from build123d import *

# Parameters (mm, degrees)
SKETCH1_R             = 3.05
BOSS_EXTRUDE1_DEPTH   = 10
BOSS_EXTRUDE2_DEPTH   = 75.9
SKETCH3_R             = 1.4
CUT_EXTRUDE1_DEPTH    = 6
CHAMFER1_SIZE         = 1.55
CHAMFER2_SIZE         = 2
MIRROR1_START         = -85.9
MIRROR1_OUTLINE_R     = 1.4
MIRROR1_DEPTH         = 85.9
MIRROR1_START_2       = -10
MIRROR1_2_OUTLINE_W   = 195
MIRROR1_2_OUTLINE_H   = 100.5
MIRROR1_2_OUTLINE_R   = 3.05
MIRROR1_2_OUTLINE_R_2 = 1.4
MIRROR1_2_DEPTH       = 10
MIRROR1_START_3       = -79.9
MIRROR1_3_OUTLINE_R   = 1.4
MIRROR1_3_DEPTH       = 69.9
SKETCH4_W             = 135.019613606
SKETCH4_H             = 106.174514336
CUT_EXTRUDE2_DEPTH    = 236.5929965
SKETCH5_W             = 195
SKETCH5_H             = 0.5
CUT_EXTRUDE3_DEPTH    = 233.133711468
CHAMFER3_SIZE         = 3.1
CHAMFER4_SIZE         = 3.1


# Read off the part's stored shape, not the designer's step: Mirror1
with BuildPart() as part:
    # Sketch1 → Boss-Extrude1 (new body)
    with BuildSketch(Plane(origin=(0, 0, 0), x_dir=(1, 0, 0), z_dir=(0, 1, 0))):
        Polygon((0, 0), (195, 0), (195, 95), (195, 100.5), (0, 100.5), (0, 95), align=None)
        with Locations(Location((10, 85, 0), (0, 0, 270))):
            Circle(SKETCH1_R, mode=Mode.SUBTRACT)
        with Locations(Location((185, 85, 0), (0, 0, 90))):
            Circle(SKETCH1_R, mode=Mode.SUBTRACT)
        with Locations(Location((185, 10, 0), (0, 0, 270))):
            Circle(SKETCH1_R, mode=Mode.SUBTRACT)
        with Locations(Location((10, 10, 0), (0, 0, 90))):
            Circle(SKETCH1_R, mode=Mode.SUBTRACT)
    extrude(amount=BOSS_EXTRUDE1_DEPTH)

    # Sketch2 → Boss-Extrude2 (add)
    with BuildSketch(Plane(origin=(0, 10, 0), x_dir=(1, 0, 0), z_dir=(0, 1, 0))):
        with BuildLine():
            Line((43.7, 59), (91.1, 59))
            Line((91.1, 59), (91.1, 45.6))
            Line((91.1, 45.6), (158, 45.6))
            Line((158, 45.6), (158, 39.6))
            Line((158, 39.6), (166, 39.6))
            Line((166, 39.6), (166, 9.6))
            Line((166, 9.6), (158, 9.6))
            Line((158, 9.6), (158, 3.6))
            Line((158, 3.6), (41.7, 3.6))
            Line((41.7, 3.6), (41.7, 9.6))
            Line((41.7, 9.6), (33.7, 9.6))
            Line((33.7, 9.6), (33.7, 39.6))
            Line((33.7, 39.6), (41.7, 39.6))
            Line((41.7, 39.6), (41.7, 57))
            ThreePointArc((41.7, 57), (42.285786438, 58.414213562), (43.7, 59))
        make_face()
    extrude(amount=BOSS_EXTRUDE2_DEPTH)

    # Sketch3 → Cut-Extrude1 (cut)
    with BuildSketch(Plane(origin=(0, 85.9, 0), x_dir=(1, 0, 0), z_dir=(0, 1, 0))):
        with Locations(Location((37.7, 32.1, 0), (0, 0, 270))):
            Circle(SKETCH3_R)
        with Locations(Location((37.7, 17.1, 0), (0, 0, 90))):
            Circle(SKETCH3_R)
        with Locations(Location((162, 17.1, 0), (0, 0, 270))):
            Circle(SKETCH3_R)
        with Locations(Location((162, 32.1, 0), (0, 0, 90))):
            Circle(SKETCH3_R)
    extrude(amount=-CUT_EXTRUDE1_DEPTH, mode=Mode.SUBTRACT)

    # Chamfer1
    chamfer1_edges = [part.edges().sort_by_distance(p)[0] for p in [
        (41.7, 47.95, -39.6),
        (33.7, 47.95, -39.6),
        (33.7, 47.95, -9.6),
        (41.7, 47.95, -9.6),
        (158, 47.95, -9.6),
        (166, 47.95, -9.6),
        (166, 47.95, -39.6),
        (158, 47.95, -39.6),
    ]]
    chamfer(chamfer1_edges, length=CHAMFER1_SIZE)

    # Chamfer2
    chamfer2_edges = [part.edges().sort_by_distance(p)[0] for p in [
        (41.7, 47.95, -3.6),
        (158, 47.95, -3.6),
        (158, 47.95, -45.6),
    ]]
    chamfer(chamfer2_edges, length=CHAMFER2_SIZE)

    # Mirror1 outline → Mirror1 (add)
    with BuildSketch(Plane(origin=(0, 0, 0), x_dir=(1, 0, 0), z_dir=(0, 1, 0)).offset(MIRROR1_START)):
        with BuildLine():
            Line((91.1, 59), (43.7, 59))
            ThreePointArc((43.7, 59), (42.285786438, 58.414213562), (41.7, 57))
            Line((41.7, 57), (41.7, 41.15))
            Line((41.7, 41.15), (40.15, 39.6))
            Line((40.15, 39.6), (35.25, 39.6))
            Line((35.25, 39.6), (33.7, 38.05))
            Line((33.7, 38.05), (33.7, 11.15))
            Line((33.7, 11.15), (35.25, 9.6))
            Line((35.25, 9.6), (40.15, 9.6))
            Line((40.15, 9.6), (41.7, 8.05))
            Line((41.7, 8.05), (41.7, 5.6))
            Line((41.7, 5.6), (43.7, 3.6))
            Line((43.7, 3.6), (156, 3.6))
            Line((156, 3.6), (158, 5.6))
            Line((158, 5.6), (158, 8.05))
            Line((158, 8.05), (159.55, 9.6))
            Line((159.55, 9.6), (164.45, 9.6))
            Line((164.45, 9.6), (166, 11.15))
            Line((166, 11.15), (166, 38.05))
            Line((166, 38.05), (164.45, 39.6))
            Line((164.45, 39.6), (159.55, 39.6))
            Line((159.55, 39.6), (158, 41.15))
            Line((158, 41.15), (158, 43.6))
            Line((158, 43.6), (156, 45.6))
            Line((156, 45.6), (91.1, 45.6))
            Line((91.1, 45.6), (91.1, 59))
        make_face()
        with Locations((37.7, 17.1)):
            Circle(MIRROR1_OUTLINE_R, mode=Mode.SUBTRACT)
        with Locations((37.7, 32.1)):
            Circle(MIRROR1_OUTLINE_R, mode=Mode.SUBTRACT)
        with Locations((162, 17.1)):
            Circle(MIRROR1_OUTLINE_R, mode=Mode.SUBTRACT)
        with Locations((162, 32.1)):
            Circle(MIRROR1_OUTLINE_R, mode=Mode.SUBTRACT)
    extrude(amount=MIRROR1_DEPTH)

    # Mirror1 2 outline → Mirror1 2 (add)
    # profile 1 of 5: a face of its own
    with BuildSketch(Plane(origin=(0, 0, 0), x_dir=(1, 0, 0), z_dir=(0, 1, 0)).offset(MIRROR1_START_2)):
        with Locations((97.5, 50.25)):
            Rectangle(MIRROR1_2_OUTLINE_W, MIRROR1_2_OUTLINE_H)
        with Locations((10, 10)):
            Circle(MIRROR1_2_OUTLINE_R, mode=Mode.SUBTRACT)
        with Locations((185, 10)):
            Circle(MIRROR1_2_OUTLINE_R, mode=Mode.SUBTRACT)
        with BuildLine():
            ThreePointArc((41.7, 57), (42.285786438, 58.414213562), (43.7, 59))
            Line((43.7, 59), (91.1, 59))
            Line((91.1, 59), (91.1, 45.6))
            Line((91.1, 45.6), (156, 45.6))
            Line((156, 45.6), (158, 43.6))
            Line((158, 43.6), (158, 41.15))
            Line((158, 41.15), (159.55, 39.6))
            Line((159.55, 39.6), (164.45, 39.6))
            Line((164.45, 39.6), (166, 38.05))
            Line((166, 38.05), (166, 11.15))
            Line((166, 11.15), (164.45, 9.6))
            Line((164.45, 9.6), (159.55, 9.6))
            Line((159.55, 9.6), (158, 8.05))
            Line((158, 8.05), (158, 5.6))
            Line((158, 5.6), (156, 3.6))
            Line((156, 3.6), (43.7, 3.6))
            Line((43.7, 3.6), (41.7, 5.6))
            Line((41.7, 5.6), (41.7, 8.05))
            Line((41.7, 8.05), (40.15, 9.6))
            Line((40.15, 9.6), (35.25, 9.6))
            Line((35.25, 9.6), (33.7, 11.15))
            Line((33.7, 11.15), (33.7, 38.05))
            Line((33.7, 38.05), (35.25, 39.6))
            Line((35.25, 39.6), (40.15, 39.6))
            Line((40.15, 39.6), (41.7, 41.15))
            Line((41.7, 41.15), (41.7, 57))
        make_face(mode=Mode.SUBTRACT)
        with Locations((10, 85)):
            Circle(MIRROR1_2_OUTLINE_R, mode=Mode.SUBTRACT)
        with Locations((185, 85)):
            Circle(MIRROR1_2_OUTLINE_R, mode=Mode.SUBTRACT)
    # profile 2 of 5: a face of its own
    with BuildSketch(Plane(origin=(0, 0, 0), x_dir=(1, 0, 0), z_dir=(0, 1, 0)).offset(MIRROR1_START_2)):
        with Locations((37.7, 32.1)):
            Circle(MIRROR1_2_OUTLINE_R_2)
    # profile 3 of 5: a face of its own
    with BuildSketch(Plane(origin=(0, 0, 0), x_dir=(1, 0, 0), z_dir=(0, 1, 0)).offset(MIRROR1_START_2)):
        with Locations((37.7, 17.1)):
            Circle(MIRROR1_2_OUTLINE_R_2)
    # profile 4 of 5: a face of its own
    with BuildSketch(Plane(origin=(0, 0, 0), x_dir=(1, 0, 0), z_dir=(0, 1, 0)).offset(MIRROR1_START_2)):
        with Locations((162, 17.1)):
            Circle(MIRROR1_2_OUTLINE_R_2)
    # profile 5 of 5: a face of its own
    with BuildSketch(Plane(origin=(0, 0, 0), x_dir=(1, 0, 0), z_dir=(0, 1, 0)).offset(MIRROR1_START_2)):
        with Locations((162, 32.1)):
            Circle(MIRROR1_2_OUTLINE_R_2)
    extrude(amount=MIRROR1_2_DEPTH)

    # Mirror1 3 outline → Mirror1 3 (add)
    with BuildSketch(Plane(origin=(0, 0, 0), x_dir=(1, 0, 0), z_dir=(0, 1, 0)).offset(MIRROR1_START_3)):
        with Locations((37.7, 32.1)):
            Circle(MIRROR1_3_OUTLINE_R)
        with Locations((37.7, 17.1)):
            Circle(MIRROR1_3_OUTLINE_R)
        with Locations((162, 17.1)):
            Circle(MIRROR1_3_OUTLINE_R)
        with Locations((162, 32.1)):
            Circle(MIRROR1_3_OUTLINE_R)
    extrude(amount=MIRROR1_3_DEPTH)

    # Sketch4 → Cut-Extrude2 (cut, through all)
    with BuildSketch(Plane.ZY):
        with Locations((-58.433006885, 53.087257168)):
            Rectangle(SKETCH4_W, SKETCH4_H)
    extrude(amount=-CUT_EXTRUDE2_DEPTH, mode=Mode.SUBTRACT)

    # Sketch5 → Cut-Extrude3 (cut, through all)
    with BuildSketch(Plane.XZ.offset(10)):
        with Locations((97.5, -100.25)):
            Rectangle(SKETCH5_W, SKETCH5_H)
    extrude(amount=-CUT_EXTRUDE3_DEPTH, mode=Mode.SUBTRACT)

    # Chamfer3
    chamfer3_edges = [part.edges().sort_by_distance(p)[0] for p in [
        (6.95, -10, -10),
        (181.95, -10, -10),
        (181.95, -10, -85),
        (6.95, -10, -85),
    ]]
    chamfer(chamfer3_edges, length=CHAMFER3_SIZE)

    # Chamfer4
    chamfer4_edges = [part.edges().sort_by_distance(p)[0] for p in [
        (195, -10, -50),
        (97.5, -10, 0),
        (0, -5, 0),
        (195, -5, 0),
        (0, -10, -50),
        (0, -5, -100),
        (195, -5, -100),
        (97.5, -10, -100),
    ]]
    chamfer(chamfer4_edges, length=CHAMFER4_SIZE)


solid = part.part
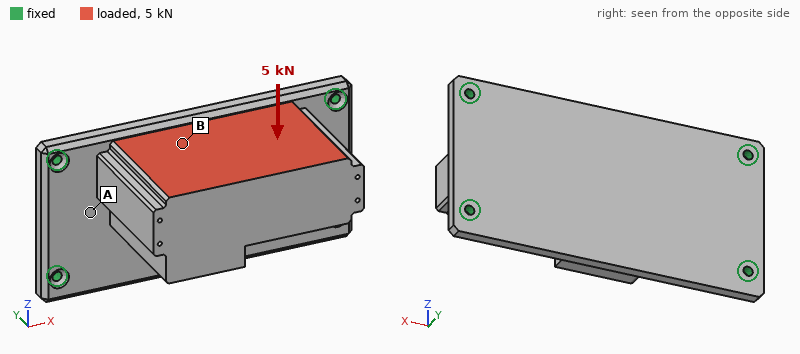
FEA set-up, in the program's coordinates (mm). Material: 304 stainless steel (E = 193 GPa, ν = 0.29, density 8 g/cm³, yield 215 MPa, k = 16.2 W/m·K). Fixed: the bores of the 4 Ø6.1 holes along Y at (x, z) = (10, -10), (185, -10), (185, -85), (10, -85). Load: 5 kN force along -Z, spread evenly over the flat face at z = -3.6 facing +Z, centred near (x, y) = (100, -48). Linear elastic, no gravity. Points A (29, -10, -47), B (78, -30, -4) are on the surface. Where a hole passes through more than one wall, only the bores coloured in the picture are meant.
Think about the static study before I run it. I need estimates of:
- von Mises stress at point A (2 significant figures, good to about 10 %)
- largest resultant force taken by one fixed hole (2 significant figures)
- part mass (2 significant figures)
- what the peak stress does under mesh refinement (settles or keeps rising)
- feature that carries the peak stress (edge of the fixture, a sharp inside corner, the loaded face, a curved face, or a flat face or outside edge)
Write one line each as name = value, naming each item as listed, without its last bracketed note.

von Mises stress at point A = 32 MPa
largest resultant force taken by one fixed hole = 2.6 kN
part mass = 5.2 kg
what the peak stress does under mesh refinement = keeps rising
feature that carries the peak stress = edge of the fixture
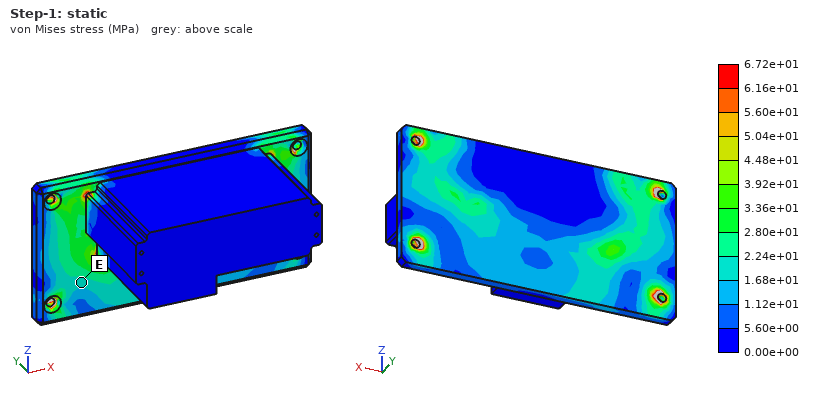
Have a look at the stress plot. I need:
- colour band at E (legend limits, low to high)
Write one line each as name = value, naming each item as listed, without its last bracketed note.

colour band at E = 1.68e+01 to 2.24e+01 MPa
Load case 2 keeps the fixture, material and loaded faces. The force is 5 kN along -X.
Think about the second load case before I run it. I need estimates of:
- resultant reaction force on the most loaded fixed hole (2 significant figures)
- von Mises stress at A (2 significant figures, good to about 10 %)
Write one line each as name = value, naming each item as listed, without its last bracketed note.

resultant reaction force on the most loaded fixed hole = 2.0 kN
von Mises stress at A = 8.3 MPa
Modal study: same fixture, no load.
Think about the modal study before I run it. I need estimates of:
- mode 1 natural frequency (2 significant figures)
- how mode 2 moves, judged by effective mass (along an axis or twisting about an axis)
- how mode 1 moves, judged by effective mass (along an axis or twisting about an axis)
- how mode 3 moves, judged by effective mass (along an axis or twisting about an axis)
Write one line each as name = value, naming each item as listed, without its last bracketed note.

mode 1 natural frequency = 840 Hz
how mode 2 moves, judged by effective mass = along Y
how mode 1 moves, judged by effective mass = along Z
how mode 3 moves, judged by effective mass = along X
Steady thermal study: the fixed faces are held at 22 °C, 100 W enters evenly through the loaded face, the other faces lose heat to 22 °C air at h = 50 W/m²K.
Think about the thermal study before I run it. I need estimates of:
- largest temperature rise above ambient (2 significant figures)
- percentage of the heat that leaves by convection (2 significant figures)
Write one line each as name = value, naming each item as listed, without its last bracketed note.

largest temperature rise above ambient = 66 K
percentage of the heat that leaves by convection = 87 %
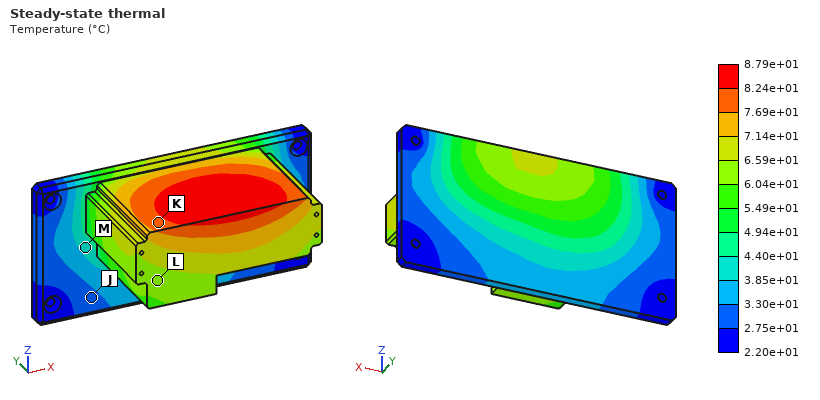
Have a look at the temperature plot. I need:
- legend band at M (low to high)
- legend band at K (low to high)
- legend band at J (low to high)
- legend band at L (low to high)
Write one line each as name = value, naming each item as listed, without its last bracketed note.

legend band at M = 3.85e+01 to 4.40e+01 °C
legend band at K = 7.69e+01 to 8.24e+01 °C
legend band at J = 2.75e+01 to 3.30e+01 °C
legend band at L = 6.04e+01 to 6.59e+01 °C
